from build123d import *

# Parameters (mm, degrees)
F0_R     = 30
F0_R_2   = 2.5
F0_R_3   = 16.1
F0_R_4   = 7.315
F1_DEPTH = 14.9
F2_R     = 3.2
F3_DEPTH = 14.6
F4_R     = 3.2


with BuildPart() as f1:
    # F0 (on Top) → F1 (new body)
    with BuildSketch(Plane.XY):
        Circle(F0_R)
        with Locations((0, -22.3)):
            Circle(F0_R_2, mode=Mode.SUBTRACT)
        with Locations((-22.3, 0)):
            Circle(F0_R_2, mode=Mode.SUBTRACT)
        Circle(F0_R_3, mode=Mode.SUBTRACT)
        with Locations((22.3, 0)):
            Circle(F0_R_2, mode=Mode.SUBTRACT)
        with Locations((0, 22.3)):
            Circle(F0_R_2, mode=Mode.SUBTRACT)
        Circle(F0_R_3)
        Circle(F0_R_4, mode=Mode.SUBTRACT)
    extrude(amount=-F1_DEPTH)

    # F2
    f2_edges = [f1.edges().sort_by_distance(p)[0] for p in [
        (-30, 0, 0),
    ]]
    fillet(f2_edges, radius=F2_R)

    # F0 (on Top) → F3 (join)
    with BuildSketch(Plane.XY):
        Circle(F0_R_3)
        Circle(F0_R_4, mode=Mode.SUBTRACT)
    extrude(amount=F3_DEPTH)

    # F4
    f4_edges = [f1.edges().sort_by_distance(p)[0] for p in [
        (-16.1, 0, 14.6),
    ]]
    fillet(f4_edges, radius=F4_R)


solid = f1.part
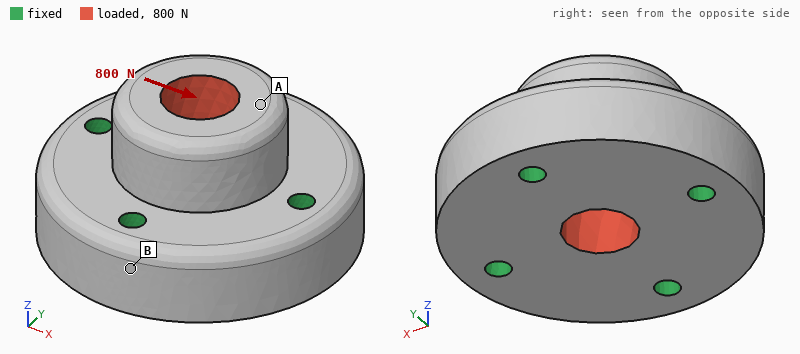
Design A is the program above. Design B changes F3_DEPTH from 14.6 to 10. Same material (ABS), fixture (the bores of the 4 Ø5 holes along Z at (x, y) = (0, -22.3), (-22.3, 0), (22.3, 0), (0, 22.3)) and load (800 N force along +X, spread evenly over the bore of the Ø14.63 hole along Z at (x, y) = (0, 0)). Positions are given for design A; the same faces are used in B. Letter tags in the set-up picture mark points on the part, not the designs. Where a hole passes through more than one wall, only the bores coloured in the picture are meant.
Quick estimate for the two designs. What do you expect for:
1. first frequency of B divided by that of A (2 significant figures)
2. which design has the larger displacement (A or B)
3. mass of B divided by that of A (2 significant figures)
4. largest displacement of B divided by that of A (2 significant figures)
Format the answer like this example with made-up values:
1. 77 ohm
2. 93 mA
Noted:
1. 1.2
2. A
3. 0.94
4. 0.72
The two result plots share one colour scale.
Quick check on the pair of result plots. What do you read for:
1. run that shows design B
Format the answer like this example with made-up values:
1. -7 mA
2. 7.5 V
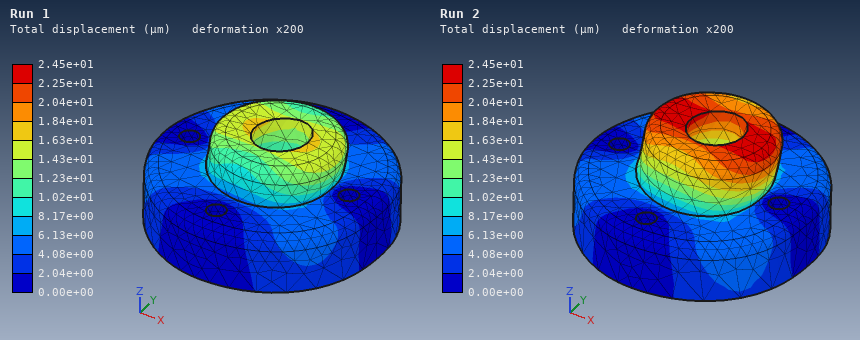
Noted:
1. Run 1
